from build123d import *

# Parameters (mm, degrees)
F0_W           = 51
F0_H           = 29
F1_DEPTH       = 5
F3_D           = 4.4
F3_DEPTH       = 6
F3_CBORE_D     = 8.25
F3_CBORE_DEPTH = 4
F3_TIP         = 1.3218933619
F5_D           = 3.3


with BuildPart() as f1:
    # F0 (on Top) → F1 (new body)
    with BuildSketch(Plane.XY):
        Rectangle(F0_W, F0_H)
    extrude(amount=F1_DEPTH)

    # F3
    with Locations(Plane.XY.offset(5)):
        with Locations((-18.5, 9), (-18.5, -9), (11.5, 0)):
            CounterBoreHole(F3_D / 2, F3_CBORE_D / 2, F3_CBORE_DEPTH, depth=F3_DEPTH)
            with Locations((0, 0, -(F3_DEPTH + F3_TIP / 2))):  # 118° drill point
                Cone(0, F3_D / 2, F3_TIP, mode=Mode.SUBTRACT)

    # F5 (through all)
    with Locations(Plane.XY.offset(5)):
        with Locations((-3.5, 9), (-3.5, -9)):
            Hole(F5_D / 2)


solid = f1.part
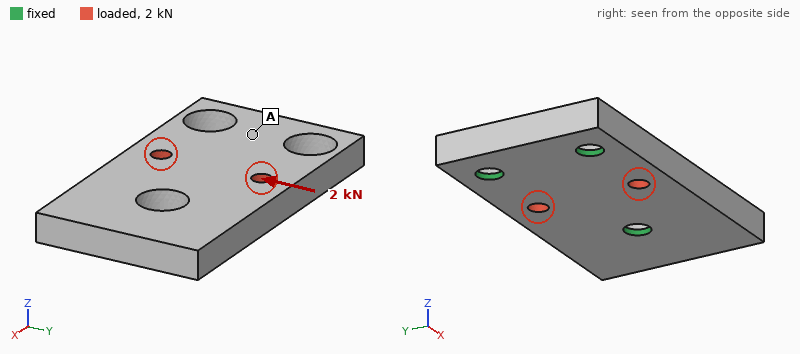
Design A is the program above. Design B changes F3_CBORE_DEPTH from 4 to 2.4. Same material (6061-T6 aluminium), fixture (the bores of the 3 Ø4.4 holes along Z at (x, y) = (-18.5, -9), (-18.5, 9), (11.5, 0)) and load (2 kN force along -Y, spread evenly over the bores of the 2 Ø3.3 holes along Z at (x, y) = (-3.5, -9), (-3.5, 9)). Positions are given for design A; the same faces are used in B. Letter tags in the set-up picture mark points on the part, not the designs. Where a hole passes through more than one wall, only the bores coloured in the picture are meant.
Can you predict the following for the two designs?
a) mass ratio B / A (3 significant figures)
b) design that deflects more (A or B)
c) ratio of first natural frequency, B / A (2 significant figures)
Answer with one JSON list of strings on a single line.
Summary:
["1.03", "A", "1.4"]
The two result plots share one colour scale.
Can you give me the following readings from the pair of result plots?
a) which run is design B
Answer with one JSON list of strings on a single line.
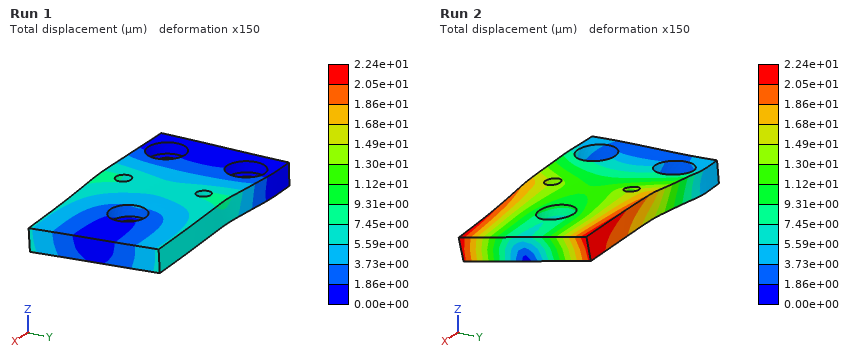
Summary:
["Run 1"]
